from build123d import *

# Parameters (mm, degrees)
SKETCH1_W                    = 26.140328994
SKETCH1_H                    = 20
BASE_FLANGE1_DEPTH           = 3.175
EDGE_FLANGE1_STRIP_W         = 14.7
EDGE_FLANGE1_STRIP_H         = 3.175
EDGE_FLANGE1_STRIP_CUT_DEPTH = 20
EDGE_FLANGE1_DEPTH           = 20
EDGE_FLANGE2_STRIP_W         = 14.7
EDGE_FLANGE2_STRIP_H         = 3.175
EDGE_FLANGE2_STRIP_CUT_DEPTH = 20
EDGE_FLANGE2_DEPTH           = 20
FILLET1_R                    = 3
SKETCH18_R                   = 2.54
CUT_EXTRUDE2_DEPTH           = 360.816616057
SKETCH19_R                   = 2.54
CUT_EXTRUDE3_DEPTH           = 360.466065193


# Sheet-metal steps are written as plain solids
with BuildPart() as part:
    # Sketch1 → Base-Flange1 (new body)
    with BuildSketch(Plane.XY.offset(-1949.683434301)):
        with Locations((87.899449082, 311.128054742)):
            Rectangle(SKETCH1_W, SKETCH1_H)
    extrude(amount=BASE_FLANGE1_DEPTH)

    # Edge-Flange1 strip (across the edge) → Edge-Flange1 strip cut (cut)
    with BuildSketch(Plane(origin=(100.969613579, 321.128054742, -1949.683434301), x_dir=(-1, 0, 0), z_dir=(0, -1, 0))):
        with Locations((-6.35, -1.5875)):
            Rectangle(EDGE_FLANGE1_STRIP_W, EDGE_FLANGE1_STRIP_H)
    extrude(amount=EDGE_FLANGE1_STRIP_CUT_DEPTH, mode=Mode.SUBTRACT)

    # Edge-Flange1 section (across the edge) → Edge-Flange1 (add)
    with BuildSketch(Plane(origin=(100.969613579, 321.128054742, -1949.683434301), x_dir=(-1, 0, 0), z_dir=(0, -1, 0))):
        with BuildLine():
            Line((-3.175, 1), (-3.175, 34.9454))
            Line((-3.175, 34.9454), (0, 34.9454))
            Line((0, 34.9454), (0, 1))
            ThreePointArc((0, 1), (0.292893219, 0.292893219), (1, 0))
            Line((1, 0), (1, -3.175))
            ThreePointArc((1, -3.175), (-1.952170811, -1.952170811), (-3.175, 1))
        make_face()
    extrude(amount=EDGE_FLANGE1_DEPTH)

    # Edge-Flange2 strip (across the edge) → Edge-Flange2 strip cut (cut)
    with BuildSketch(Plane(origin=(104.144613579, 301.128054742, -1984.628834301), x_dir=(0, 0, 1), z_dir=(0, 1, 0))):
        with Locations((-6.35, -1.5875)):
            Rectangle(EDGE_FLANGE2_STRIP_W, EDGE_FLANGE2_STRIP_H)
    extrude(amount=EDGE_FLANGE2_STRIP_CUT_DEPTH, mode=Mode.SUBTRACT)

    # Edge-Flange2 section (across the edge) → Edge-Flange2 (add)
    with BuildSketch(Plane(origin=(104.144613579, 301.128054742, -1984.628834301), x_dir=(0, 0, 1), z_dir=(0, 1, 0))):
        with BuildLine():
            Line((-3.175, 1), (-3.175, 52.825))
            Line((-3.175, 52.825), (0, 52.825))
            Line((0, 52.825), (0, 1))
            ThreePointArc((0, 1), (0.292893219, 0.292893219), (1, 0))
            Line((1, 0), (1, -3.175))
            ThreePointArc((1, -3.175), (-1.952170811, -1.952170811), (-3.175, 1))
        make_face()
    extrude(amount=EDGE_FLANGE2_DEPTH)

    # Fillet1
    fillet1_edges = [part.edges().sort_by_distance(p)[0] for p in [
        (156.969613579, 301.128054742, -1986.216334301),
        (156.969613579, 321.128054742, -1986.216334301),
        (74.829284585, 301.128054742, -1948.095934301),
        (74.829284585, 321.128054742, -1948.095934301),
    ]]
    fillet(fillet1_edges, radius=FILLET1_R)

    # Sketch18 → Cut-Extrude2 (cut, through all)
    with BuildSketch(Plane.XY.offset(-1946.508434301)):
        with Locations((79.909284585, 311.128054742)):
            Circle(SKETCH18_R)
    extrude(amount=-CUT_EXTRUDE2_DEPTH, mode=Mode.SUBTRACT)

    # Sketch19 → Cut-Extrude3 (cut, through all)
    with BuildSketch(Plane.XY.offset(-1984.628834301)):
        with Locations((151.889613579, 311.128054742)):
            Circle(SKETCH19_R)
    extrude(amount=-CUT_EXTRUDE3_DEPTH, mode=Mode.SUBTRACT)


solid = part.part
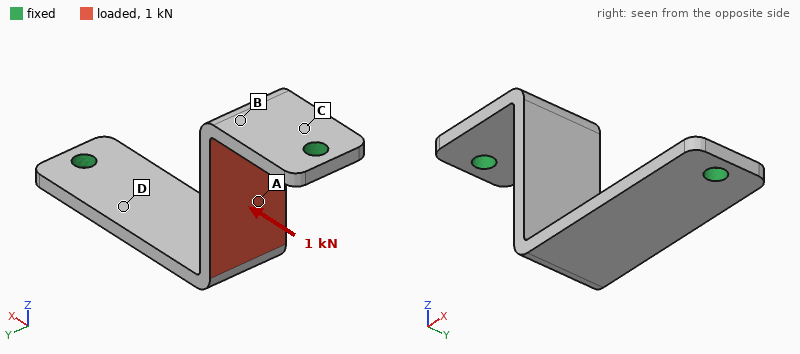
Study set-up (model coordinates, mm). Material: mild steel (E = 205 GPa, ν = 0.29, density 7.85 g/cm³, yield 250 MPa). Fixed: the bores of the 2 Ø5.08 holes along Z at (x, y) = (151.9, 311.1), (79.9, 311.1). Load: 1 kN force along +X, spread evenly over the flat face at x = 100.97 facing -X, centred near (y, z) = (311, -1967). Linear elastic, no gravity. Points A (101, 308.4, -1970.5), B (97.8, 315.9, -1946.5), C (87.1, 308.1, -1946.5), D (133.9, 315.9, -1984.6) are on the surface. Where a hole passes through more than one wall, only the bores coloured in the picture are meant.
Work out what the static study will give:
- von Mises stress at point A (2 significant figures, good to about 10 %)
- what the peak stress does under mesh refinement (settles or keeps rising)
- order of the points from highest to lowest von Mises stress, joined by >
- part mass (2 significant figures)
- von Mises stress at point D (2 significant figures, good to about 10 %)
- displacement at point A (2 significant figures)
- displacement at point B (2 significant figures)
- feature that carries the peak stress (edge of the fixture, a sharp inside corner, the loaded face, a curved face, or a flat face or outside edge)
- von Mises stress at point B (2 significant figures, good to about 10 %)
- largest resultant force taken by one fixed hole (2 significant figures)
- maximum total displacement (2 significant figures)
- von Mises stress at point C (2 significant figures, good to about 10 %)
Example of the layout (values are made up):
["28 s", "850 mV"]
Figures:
["100 MPa", "keeps rising", "A > C > B > D", "58 g", "22 MPa", "65 µm", "28 µm", "edge of the fixture", "38 MPa", "510 N", "68 µm", "50 MPa"]
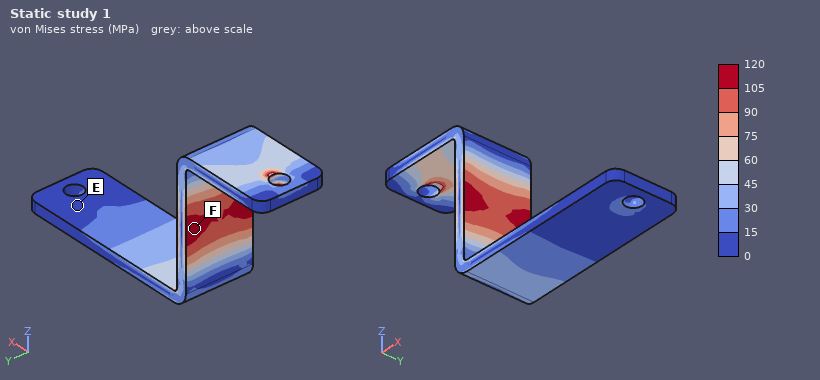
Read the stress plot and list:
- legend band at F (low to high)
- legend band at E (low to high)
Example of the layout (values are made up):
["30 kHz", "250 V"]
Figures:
["105 to 120 MPa", "0 to 15 MPa"]
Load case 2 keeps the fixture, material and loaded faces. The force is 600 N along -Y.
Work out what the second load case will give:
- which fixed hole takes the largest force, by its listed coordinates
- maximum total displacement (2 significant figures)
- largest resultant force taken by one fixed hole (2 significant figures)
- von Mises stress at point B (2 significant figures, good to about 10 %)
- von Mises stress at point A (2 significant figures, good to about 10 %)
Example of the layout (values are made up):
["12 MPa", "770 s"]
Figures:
["(79.9, 311.1)", "57 µm", "330 N", "16 MPa", "18 MPa"]
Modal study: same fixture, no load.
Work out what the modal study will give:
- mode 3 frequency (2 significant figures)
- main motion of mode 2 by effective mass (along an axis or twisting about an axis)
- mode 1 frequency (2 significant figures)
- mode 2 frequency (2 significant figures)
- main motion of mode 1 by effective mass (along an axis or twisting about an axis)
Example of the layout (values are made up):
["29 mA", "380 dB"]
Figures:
["5500 Hz", "along Y", "2400 Hz", "3200 Hz", "along Z"]
